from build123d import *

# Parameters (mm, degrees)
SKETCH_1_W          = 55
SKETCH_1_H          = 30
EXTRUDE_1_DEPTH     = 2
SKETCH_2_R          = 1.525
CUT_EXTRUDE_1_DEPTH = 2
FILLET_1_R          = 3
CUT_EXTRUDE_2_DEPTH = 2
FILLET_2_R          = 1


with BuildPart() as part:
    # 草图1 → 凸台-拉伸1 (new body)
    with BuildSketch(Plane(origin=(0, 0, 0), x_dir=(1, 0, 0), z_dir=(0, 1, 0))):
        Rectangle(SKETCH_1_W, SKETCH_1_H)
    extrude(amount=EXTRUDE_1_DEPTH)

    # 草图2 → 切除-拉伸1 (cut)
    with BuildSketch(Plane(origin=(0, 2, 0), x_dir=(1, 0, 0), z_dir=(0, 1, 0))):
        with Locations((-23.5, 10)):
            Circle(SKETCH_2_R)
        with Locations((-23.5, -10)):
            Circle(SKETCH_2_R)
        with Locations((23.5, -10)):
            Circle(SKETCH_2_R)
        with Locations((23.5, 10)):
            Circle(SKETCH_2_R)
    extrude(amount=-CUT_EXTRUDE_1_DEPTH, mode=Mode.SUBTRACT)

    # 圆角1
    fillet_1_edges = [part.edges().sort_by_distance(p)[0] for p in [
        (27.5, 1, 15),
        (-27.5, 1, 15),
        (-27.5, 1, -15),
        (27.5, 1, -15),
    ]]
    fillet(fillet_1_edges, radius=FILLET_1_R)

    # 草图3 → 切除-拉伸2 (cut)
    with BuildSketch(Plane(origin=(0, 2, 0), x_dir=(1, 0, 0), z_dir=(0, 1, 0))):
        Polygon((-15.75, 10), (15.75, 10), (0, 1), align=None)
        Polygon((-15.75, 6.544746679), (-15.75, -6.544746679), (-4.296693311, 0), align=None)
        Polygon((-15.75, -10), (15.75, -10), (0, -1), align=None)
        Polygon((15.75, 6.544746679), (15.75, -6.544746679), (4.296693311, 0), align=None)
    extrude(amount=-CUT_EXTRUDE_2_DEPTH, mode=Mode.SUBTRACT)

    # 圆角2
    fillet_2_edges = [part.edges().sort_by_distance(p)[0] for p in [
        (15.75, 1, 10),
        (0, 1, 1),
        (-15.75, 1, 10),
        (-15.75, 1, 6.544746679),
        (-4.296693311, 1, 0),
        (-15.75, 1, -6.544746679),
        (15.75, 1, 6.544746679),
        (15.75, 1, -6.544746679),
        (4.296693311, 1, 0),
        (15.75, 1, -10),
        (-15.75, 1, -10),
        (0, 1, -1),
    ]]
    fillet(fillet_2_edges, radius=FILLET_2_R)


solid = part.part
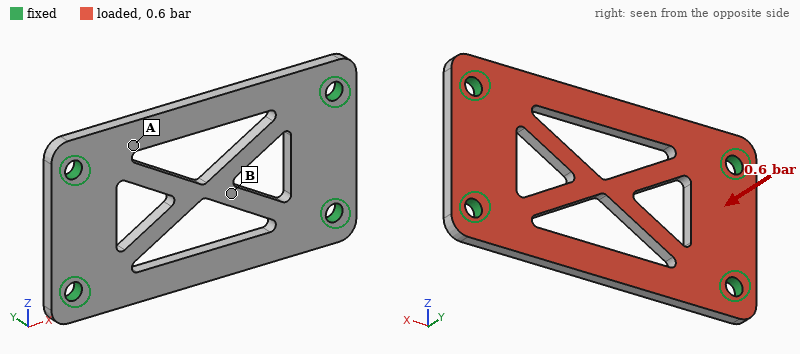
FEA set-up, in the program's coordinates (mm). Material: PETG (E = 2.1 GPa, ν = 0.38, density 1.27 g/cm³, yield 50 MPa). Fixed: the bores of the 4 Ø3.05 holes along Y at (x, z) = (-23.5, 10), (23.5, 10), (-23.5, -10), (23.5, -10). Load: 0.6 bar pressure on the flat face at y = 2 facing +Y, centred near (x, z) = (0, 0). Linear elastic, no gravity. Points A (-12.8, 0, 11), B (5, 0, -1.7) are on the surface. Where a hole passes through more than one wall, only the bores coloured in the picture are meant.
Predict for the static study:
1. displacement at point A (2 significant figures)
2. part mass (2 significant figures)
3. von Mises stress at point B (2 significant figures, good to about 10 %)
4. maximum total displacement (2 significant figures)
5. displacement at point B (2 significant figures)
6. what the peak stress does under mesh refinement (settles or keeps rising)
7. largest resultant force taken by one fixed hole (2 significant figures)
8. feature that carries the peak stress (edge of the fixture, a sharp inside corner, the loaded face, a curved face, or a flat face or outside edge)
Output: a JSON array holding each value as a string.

["0.19 mm", "3.0 g", "4.7 MPa", "0.48 mm", "0.42 mm", "keeps rising", "18 N", "edge of the fixture"]
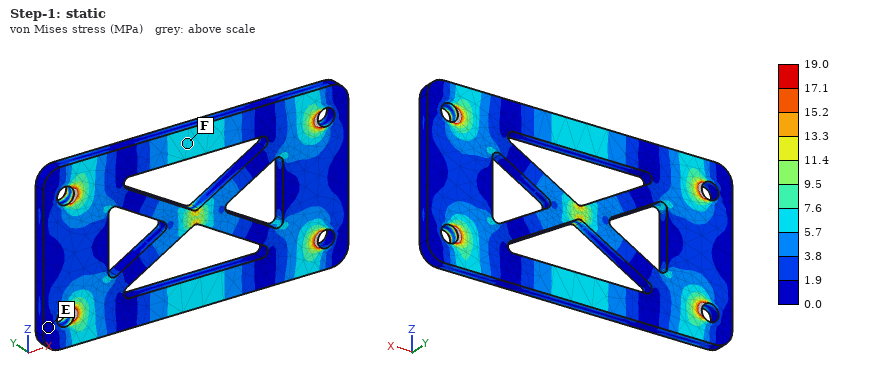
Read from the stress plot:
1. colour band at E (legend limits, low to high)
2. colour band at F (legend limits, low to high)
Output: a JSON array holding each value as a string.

["0.0 to 1.9 MPa", "5.7 to 7.6 MPa"]
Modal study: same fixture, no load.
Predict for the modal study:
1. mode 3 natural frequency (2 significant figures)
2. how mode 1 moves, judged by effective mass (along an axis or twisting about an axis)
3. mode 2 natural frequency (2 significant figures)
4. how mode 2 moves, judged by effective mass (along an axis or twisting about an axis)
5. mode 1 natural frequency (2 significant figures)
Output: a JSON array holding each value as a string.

["2100 Hz", "along Y", "1600 Hz", "twisting about X", "1400 Hz"]
